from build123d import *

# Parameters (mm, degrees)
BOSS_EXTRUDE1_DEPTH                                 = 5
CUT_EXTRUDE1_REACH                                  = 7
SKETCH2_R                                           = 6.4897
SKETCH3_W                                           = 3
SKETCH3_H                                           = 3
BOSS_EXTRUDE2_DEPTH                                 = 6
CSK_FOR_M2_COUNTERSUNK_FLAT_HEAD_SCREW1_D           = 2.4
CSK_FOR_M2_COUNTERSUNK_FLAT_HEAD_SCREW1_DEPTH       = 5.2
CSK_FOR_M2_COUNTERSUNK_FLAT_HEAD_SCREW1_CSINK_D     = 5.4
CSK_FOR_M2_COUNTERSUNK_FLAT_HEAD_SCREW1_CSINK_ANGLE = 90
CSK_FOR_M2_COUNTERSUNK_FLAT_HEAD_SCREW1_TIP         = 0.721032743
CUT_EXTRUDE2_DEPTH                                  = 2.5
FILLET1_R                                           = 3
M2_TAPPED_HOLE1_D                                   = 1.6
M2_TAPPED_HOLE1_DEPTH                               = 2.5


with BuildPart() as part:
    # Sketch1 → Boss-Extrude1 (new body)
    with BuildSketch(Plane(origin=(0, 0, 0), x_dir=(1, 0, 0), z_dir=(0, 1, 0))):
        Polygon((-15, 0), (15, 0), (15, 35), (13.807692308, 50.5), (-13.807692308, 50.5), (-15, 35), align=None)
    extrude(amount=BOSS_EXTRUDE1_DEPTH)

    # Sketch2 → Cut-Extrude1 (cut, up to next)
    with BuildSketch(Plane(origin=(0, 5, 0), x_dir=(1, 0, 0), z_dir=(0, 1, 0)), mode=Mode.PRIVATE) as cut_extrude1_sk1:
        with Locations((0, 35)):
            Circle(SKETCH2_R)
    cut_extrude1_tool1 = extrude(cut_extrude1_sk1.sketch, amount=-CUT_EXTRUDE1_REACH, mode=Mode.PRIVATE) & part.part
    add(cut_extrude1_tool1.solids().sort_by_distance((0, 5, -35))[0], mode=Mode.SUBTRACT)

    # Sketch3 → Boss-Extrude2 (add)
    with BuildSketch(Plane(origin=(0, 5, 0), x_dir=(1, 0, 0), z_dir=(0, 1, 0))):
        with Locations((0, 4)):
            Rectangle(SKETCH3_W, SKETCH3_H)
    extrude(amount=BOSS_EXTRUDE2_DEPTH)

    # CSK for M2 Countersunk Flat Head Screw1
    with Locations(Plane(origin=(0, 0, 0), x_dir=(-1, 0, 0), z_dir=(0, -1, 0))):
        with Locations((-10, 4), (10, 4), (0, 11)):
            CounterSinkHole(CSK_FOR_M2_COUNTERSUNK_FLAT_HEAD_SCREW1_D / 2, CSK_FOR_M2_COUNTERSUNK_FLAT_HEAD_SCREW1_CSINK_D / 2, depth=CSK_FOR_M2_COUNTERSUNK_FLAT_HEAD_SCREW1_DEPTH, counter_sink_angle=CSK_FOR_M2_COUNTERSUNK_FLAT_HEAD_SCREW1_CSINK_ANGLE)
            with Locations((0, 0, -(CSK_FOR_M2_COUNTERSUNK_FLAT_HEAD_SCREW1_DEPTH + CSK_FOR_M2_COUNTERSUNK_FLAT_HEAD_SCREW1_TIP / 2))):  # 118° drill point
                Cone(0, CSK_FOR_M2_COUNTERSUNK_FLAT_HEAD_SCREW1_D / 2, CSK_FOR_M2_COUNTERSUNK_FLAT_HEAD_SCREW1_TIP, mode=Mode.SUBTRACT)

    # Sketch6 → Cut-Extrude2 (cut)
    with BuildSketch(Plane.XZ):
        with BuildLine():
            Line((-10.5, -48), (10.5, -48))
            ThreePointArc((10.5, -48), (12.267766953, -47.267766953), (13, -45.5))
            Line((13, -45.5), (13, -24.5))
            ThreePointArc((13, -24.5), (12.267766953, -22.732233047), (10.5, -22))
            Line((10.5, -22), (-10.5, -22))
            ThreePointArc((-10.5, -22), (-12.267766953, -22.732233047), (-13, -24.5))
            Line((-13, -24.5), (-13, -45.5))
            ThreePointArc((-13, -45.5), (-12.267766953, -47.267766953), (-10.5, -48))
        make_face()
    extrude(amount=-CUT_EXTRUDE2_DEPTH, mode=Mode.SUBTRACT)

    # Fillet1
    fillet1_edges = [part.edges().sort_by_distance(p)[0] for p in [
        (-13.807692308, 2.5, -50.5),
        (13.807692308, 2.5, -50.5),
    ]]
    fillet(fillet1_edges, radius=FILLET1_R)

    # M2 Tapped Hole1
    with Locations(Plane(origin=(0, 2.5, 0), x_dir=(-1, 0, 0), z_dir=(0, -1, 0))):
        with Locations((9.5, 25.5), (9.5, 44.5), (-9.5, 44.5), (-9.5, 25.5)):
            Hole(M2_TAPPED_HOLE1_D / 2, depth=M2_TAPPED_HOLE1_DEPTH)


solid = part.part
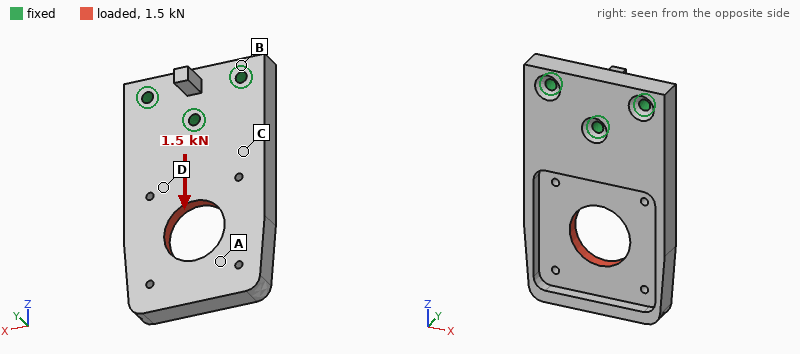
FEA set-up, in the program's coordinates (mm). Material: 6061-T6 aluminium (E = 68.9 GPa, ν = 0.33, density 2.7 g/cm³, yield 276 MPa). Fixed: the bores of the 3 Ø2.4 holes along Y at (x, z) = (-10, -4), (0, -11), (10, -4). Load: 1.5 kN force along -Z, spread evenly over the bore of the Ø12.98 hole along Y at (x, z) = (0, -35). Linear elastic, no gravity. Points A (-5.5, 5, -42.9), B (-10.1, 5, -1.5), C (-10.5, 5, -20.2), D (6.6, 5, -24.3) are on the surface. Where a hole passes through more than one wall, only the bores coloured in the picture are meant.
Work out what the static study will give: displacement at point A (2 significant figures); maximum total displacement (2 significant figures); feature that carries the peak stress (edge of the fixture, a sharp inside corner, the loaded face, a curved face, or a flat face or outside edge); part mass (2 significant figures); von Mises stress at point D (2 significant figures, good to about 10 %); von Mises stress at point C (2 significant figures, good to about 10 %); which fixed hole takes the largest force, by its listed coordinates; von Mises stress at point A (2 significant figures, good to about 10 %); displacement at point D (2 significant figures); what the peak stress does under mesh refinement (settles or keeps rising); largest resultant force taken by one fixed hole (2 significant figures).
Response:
41 µm
56 µm
edge of the fixture
15 g
28 MPa
24 MPa
(0, -11)
15 MPa
12 µm
keeps rising
650 N
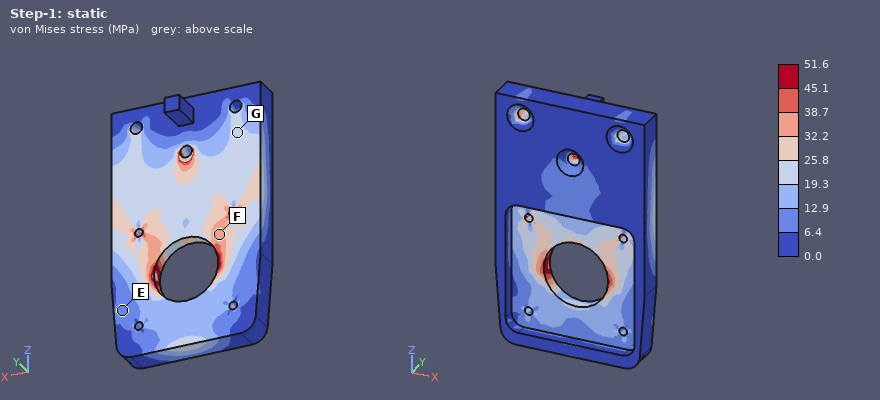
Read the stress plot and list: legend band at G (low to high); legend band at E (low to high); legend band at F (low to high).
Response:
19.3 to 25.8 MPa
6.4 to 12.9 MPa
32.2 to 38.7 MPa
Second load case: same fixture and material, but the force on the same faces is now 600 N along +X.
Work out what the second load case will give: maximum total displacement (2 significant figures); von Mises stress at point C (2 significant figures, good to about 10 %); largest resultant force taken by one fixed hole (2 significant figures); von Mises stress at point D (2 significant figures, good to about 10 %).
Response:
35 µm
14 MPa
670 N
11 MPa
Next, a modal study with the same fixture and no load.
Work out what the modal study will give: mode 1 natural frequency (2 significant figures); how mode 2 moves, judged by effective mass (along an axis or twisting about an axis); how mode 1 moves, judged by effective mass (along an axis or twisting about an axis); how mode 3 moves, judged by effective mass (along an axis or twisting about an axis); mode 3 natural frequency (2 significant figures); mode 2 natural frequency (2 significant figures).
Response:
2300 Hz
twisting about Z
along Y
along X
9600 Hz
4600 Hz
